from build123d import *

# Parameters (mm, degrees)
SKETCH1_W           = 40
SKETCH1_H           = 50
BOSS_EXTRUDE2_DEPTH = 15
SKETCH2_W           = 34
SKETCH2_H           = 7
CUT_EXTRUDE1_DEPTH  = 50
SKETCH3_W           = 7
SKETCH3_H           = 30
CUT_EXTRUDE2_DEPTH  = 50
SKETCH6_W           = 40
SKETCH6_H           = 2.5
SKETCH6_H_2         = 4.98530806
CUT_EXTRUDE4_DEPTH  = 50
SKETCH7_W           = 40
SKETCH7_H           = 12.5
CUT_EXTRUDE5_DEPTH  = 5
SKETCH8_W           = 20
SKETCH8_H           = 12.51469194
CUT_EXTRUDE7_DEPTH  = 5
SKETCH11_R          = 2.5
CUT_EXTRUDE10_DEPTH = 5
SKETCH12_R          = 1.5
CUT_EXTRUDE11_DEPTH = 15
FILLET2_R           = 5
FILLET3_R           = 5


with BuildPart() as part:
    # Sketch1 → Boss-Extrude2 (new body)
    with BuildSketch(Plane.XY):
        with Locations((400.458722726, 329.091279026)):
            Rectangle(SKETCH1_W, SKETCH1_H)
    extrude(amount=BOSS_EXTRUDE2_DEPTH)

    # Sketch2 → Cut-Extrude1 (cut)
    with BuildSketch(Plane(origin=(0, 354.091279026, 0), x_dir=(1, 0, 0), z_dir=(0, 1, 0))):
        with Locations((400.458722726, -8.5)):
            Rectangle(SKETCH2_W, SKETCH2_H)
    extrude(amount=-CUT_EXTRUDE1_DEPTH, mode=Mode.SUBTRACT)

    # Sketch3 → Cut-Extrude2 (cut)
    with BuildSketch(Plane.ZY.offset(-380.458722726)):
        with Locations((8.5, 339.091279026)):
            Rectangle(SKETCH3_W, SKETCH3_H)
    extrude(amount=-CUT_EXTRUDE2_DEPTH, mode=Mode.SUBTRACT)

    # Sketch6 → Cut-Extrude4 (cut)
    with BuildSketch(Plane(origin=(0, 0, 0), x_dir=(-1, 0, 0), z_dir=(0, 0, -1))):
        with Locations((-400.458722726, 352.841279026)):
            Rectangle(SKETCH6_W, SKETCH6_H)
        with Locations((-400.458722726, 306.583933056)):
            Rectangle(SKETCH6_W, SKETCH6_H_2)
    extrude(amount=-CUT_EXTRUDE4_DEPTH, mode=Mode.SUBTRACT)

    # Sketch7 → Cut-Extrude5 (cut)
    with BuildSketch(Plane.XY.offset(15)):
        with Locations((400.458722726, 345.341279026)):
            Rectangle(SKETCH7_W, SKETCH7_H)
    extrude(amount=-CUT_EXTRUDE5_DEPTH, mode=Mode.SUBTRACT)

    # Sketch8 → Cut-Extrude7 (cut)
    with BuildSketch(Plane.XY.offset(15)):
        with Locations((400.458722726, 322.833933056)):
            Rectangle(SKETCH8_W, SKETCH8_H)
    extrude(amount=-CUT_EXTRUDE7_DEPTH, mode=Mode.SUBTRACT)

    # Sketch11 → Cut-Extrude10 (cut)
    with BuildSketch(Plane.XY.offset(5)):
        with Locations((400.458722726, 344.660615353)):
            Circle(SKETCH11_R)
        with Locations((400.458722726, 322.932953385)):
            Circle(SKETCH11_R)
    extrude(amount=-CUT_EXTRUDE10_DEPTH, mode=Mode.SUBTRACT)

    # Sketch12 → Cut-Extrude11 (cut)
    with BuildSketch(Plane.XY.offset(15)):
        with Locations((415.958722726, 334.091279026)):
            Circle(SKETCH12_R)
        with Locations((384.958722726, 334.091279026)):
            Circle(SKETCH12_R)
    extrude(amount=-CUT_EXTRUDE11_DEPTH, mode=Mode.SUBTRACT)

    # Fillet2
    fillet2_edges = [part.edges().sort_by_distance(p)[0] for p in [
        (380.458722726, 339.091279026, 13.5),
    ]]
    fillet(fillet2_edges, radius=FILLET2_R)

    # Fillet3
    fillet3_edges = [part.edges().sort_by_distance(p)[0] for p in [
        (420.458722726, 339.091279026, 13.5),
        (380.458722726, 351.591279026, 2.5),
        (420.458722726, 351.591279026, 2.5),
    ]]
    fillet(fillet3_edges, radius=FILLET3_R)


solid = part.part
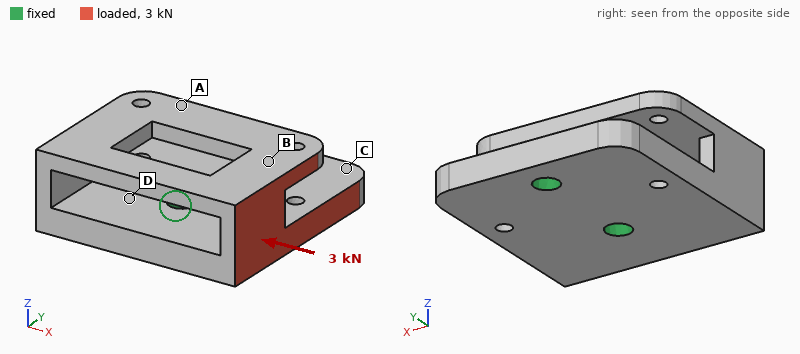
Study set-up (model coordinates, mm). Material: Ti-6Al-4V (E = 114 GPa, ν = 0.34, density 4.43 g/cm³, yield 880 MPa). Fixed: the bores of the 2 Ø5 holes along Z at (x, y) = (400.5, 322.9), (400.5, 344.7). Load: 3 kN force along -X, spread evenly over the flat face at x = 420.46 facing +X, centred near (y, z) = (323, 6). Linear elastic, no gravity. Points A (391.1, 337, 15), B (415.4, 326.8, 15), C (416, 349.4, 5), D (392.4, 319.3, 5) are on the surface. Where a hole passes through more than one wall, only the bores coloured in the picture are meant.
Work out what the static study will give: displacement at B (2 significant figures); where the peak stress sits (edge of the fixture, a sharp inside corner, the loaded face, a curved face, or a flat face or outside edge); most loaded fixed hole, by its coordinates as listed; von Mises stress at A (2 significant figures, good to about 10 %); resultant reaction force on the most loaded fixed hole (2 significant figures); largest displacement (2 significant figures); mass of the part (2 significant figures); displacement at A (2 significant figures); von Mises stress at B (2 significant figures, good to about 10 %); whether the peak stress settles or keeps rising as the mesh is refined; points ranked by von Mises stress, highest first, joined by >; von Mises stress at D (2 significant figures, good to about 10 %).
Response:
64 µm
edge of the fixture
(400.5, 322.9)
20 MPa
2.8 kN
74 µm
51 g
61 µm
38 MPa
keeps rising
D > B > A > C
52 MPa
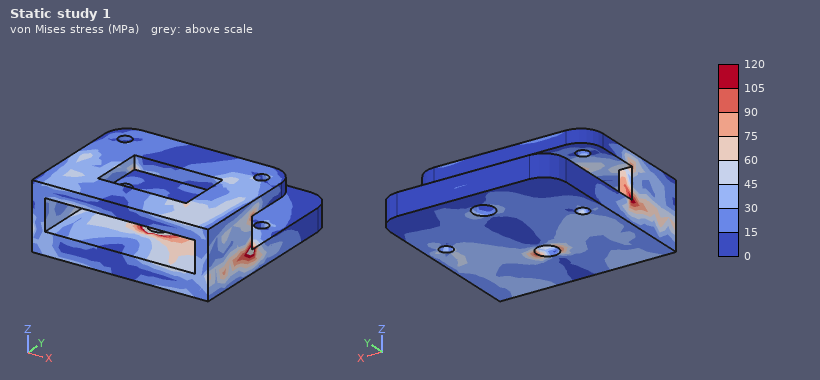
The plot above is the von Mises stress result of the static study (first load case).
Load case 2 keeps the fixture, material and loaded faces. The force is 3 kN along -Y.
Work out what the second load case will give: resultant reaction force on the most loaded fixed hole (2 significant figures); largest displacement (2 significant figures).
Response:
2.9 kN
0.10 mm
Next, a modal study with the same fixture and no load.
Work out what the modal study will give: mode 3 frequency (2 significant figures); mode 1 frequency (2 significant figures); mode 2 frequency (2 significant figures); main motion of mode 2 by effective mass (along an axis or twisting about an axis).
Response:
6200 Hz
3900 Hz
4900 Hz
along X
